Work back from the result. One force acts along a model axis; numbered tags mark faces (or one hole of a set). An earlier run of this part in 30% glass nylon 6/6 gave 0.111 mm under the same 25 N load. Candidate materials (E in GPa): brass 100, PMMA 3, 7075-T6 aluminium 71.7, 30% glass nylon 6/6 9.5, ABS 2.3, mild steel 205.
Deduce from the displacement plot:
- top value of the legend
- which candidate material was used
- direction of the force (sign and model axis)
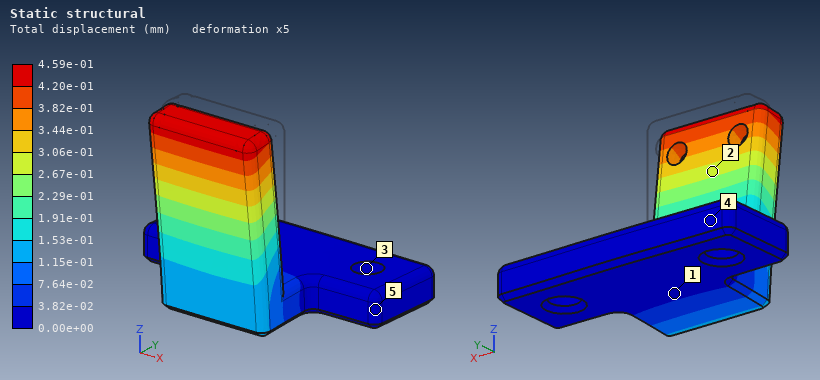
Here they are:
4.59e-01 mm
ABS
-Y
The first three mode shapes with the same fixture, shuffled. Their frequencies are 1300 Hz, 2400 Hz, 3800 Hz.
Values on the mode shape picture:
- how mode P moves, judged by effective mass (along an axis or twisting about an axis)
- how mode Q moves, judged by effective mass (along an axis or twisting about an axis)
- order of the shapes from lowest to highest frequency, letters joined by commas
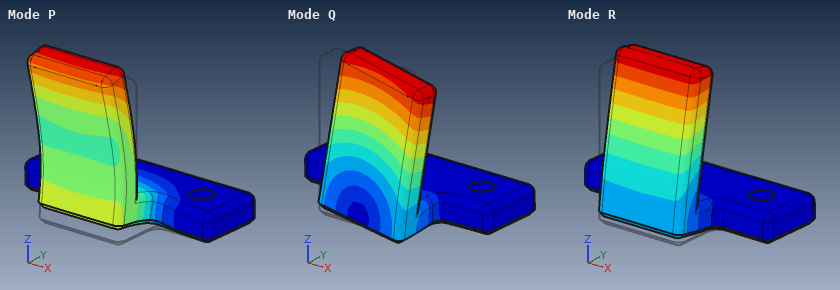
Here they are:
along Z
along X
R, Q, P
